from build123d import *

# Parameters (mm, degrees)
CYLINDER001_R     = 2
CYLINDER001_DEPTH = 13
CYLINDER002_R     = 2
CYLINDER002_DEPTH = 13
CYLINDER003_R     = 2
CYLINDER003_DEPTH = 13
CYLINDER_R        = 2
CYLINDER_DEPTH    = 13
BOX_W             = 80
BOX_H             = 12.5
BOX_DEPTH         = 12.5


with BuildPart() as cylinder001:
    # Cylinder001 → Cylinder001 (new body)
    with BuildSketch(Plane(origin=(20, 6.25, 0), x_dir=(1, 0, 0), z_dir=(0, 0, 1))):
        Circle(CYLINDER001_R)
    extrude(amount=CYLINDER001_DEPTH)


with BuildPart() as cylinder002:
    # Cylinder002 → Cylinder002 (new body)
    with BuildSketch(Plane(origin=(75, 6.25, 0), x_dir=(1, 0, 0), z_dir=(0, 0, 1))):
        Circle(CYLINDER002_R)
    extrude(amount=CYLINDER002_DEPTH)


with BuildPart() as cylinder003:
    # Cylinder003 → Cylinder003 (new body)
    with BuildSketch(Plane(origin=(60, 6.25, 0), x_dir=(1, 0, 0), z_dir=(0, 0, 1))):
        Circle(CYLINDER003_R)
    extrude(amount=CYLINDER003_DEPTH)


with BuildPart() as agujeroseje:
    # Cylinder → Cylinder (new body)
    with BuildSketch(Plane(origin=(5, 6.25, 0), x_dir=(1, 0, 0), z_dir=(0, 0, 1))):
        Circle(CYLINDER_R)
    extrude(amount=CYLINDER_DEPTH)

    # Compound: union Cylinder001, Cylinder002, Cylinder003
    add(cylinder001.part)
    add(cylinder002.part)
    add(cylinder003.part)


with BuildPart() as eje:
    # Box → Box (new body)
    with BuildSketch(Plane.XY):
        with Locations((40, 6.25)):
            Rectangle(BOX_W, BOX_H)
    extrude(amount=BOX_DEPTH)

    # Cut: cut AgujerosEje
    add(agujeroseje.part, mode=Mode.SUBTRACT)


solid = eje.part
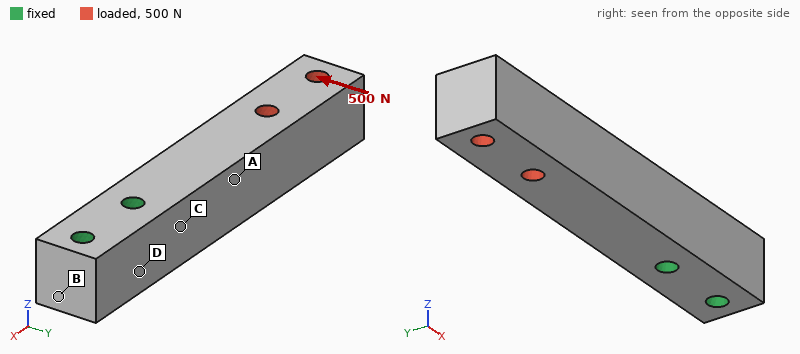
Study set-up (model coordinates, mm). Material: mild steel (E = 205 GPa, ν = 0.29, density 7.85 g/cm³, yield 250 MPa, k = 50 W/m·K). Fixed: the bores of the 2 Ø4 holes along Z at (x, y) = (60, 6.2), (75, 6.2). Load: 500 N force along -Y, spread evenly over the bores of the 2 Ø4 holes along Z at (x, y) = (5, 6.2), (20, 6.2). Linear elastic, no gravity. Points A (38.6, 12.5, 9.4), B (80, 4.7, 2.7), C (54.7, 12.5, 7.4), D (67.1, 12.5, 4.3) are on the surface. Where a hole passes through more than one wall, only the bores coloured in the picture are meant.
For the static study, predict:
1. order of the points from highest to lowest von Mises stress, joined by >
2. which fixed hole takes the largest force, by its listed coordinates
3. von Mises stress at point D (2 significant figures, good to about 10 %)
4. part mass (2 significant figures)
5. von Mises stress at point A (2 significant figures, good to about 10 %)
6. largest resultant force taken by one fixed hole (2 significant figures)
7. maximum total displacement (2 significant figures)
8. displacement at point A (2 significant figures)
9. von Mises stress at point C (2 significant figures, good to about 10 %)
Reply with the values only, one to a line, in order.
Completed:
C > A > D > B
(60, 6.2)
18 MPa
93 g
40 MPa
1.3 kN
75 µm
18 µm
64 MPa
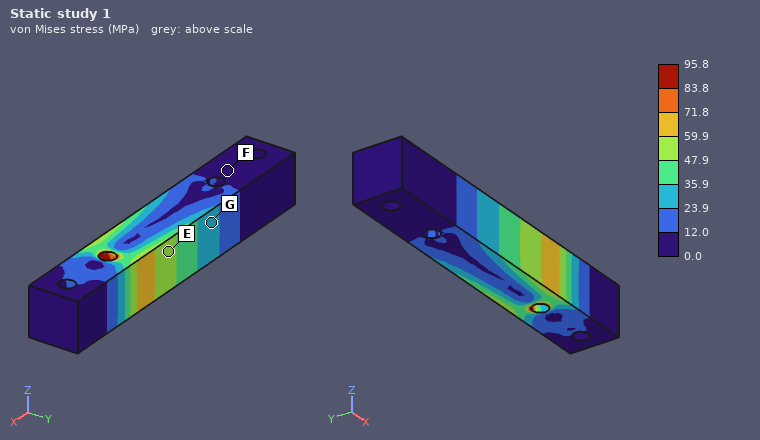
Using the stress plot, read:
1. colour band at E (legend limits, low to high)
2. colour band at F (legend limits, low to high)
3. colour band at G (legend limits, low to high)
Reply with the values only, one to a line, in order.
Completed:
47.9 to 59.9 MPa
0.0 to 12.0 MPa
23.9 to 35.9 MPa
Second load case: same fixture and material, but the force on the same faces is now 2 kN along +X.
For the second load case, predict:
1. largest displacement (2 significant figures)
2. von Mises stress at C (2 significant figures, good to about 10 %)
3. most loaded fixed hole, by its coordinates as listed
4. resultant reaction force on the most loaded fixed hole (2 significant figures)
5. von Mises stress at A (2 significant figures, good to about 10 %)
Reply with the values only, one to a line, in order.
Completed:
3.4 µm
9.3 MPa
(60, 6.2)
1.8 kN
13 MPa
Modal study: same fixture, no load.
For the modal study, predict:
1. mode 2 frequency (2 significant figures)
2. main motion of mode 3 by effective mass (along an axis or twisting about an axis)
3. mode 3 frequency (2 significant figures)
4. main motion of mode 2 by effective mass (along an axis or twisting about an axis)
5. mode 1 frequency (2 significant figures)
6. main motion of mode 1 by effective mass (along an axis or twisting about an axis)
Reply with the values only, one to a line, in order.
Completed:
2900 Hz
twisting about X
12 kHz
along Z
2600 Hz
along Y
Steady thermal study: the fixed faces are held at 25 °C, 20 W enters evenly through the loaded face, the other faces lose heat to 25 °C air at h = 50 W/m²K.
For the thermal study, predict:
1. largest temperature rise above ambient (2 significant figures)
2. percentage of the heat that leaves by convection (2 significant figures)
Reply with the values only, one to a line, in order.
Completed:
87 K
38 %
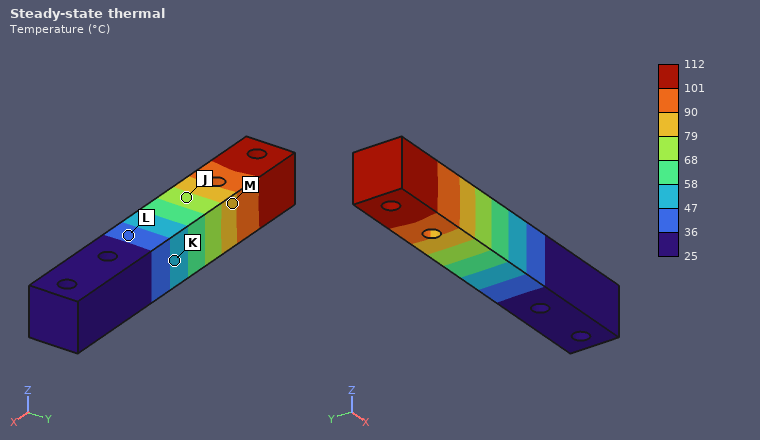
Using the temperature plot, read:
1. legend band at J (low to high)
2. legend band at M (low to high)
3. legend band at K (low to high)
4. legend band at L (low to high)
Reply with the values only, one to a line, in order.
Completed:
68 to 79 °C
79 to 90 °C
47 to 58 °C
36 to 47 °C
